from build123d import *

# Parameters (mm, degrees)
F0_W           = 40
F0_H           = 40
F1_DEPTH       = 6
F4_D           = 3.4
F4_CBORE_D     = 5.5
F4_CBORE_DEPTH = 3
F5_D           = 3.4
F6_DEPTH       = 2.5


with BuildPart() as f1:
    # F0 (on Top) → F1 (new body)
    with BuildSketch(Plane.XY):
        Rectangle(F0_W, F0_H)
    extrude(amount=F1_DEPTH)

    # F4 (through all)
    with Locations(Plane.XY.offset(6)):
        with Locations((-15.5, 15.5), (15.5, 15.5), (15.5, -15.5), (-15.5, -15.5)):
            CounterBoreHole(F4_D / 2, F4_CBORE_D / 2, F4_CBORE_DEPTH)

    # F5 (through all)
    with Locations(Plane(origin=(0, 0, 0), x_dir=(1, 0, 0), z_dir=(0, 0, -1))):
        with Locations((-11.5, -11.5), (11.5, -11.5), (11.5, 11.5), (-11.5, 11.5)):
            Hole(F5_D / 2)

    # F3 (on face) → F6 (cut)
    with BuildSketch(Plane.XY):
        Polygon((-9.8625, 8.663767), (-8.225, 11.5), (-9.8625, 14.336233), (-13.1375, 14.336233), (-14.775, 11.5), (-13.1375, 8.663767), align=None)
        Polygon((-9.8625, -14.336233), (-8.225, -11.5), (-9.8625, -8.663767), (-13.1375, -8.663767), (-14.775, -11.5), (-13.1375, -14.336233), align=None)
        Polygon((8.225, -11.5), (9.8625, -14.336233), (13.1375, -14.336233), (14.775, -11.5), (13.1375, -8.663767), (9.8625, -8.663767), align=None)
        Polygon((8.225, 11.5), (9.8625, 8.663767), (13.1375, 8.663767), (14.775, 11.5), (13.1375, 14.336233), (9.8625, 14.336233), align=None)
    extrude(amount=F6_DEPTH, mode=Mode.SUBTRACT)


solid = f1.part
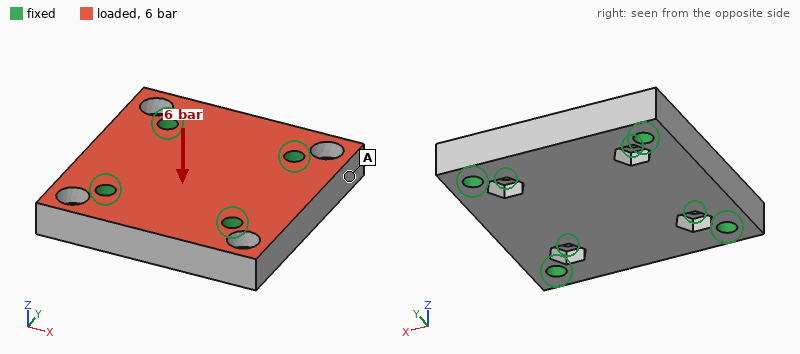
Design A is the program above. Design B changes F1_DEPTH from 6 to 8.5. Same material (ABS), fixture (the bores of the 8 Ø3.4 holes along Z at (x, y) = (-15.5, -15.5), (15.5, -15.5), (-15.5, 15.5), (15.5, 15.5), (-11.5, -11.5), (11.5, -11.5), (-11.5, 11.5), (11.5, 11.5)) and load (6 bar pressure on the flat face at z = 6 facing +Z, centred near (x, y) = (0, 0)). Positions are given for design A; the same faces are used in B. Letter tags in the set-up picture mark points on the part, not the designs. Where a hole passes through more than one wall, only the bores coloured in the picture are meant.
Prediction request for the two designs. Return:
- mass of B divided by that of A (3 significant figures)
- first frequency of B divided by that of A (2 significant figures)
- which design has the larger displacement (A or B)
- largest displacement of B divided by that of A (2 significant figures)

1.42
1.2
A
0.47
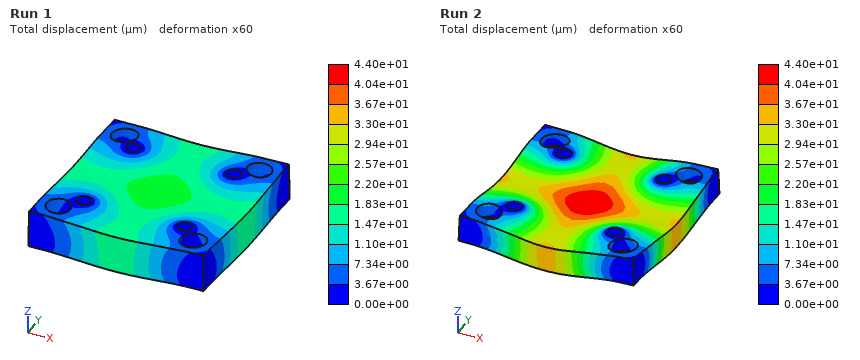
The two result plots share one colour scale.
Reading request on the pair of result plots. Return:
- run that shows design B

Run 1
